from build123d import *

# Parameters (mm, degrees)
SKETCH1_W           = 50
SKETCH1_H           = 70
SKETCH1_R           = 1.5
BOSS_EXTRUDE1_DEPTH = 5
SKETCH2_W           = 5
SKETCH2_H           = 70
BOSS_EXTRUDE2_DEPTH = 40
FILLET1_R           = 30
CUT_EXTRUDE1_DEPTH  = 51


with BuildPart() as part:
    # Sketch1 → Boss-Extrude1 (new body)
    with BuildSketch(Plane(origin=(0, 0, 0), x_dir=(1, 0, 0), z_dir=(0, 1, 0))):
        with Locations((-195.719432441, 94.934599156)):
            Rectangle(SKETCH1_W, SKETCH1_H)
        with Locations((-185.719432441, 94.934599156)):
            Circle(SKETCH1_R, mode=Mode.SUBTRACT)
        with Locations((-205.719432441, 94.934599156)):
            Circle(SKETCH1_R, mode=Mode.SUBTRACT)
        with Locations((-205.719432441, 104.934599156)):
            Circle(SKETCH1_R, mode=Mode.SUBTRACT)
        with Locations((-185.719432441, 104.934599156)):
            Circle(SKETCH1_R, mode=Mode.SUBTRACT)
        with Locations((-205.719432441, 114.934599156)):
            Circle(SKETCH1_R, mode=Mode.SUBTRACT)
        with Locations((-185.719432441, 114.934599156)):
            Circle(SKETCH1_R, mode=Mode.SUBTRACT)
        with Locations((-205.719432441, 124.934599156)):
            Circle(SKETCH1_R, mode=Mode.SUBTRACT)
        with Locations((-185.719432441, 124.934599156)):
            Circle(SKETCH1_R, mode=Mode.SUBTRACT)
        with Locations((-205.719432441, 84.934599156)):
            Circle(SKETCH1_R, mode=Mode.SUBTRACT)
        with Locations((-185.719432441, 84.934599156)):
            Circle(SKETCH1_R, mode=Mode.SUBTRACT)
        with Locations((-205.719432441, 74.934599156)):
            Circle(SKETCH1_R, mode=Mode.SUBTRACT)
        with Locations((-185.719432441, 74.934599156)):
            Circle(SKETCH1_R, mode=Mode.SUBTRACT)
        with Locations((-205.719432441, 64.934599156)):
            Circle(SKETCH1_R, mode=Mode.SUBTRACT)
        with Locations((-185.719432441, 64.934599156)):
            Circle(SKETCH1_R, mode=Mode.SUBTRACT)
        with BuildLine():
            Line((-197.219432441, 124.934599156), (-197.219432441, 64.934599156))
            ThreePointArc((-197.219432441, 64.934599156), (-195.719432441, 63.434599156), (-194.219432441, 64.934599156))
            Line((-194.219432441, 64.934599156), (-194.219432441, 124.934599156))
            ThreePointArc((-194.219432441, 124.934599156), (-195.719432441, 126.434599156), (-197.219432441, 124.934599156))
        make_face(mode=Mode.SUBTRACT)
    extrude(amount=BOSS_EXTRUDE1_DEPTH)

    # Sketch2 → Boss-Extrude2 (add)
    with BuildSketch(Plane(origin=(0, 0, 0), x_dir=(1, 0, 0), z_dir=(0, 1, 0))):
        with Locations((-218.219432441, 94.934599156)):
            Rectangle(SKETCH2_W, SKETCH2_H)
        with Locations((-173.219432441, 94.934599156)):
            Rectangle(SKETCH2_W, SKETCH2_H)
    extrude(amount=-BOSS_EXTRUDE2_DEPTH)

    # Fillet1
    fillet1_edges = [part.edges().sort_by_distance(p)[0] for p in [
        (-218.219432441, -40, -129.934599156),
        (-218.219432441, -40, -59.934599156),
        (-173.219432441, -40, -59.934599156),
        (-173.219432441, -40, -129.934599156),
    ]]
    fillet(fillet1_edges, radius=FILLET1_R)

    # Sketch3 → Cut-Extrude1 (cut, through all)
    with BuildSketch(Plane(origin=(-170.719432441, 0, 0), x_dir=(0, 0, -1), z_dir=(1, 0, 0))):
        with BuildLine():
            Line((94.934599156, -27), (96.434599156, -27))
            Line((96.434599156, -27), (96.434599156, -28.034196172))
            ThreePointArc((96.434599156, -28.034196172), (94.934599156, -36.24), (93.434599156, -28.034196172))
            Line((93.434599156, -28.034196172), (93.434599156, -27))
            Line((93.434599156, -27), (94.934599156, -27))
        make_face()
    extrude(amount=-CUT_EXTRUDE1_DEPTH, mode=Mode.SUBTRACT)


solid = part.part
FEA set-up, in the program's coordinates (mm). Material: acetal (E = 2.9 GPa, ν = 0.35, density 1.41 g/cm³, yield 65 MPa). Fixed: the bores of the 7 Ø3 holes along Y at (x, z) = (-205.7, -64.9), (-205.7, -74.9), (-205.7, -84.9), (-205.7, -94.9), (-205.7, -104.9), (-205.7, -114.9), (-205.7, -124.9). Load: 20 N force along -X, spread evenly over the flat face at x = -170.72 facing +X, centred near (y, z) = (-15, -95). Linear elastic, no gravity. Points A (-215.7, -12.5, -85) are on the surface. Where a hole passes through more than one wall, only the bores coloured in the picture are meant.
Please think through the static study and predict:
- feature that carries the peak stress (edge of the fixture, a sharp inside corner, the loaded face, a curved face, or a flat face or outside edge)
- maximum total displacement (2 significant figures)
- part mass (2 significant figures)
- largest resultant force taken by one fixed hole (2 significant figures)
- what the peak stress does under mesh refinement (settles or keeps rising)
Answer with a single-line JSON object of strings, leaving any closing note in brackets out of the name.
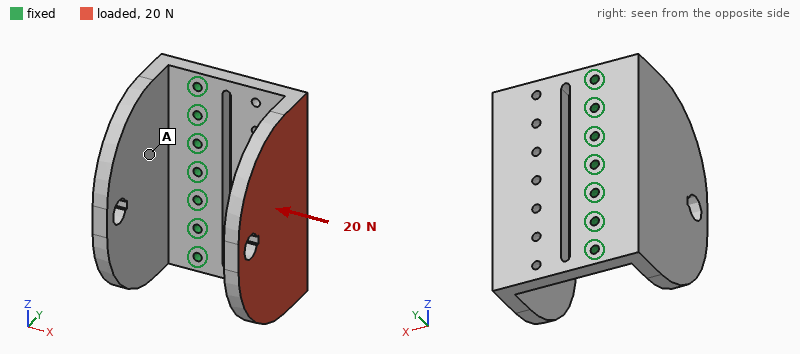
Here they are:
{"feature that carries the peak stress": "a sharp inside corner", "maximum total displacement": "1.1 mm", "part mass": "56 g", "largest resultant force taken by one fixed hole": "12 N", "what the peak stress does under mesh refinement": "keeps rising"}
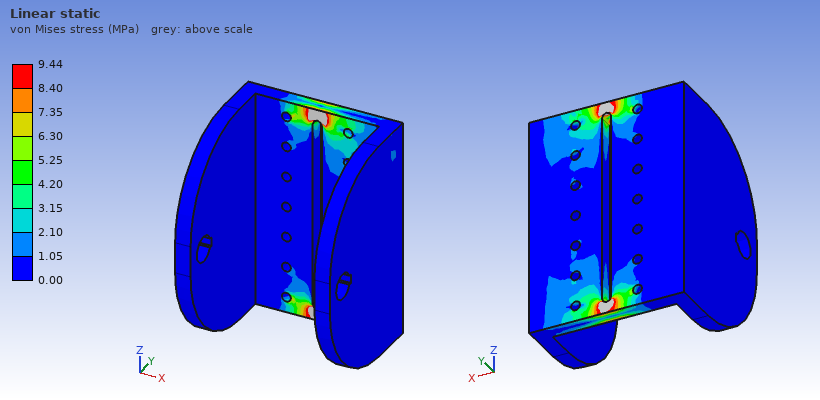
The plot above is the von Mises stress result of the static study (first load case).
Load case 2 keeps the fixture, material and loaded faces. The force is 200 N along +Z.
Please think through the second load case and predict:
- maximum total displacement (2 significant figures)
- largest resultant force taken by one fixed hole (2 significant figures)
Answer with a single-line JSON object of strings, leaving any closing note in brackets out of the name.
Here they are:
{"maximum total displacement": "0.95 mm", "largest resultant force taken by one fixed hole": "150 N"}
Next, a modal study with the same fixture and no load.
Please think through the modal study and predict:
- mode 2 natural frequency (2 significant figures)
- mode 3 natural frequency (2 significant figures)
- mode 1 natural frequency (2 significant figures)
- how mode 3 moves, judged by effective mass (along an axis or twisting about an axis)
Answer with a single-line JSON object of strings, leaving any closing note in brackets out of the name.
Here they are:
{"mode 2 natural frequency": "500 Hz", "mode 3 natural frequency": "570 Hz", "mode 1 natural frequency": "150 Hz", "how mode 3 moves, judged by effective mass": "along X"}
